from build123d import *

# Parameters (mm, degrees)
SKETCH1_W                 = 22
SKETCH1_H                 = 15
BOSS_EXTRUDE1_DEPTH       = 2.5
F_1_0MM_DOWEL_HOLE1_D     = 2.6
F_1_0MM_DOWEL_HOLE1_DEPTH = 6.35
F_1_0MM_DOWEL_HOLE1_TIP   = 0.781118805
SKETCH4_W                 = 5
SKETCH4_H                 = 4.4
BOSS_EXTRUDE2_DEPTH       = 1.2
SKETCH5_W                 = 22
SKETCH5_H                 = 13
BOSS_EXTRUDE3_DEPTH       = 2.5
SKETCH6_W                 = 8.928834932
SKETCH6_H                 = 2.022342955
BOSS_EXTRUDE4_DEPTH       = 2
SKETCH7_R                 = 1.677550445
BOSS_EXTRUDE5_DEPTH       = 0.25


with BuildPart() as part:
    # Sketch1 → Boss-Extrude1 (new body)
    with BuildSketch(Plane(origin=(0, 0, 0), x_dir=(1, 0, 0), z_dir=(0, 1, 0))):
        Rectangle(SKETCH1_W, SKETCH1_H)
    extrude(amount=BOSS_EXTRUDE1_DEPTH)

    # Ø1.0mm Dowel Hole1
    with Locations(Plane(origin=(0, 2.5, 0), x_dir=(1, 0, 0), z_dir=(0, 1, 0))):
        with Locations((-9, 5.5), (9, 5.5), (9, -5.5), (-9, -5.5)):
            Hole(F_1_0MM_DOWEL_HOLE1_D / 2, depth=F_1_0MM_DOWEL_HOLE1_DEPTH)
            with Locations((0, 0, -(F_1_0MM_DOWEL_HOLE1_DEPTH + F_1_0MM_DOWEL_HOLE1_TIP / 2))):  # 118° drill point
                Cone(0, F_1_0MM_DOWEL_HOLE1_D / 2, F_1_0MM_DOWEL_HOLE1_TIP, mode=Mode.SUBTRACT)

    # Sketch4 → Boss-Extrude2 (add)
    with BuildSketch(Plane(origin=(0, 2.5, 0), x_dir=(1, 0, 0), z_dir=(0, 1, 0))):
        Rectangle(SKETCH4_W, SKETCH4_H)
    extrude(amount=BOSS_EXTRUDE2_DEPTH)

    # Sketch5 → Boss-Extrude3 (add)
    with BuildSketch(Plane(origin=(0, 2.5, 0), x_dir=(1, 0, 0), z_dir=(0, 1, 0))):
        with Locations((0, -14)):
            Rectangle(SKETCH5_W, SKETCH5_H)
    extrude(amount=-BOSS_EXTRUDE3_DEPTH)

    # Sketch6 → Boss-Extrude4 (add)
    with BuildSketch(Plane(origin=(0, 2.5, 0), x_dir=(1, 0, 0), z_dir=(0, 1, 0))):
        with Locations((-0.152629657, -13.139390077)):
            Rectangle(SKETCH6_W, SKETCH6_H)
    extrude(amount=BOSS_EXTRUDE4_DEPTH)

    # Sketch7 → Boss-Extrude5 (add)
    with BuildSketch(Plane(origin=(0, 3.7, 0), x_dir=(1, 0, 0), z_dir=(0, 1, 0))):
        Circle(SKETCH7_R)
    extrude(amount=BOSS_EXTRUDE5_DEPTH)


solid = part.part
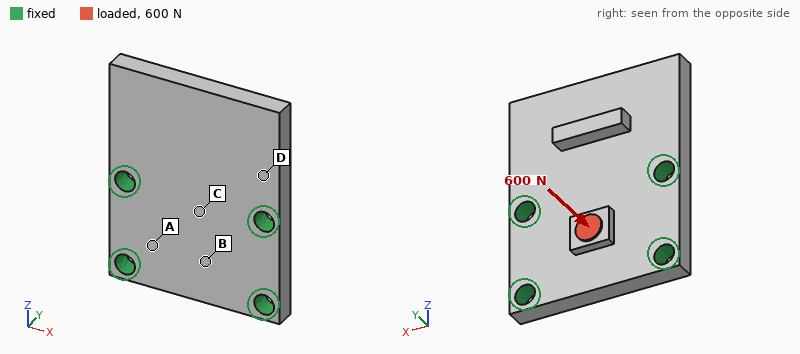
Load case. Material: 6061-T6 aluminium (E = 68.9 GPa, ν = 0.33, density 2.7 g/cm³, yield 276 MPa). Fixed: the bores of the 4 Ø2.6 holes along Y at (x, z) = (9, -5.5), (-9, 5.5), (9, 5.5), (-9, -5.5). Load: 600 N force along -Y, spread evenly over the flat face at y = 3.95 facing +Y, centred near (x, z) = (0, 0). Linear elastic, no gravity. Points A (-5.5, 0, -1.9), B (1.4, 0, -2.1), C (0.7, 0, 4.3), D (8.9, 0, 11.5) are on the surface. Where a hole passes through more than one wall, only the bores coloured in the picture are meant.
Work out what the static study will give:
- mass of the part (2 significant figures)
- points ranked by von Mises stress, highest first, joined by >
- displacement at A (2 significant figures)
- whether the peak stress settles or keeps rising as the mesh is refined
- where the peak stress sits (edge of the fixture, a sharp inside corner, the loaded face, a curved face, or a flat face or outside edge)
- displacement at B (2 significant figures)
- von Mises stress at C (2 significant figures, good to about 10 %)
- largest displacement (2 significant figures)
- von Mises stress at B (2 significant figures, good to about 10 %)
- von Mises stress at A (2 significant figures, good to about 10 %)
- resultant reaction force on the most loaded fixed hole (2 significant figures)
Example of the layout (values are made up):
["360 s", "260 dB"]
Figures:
["4.2 g", "B > C > A > D", "6.7 µm", "keeps rising", "edge of the fixture", "13 µm", "38 MPa", "15 µm", "55 MPa", "21 MPa", "150 N"]
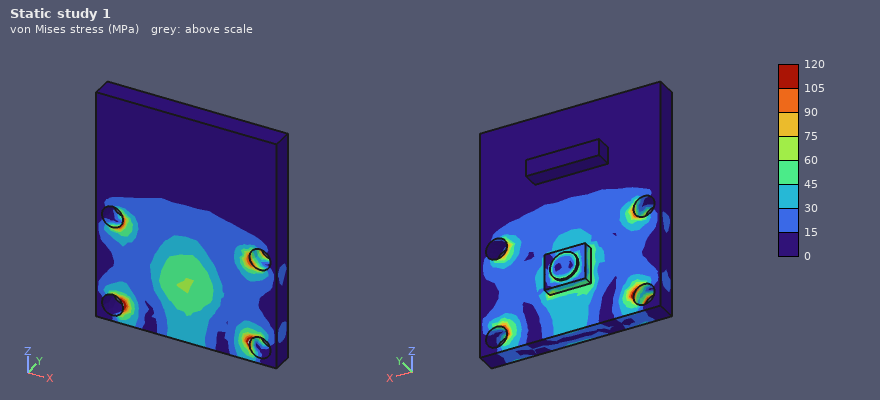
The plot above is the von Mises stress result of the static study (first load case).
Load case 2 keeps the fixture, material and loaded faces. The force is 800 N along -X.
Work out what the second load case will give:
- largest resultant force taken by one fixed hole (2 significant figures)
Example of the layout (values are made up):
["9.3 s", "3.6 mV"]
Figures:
["230 N"]
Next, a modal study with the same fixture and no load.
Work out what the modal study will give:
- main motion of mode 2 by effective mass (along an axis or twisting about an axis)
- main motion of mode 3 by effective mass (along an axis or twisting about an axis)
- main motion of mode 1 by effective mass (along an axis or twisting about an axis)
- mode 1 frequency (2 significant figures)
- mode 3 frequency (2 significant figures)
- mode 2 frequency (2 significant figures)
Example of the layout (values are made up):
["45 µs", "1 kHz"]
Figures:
["twisting about Z", "along Y", "along Y", "8500 Hz", "35 kHz", "17 kHz"]
